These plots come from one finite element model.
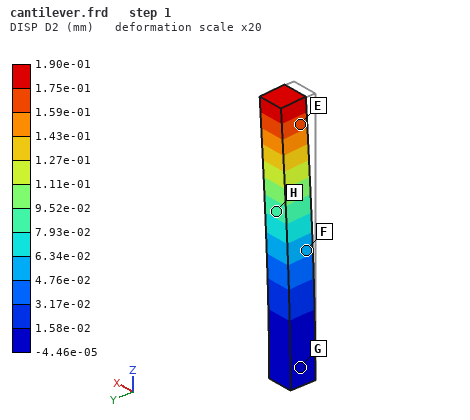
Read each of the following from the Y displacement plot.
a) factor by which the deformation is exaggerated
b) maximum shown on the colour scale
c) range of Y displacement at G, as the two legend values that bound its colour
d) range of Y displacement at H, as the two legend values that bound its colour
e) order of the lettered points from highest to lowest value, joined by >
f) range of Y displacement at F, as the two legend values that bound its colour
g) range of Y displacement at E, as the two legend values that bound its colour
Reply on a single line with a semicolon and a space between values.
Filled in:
20; 1.90e-01 mm; -4.46e-05 to 1.58e-02 mm; 7.93e-02 to 9.52e-02 mm; E > H > F > G; 4.76e-02 to 6.34e-02 mm; 1.59e-01 to 1.75e-01 mm
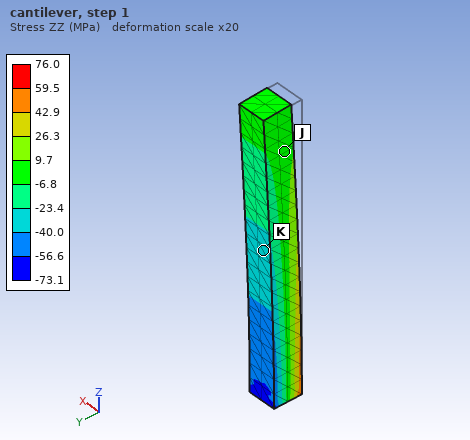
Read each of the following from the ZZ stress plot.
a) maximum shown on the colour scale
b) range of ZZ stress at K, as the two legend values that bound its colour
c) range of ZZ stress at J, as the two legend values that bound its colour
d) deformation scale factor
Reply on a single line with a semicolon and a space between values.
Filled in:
76.0 MPa; -40.0 to -23.4 MPa; -6.8 to 9.7 MPa; 20
